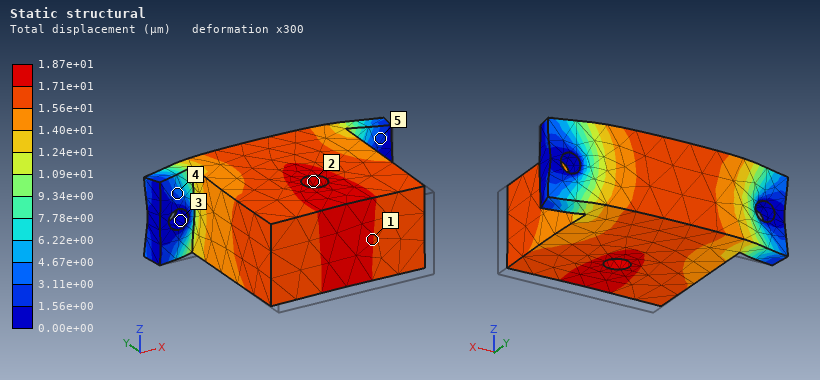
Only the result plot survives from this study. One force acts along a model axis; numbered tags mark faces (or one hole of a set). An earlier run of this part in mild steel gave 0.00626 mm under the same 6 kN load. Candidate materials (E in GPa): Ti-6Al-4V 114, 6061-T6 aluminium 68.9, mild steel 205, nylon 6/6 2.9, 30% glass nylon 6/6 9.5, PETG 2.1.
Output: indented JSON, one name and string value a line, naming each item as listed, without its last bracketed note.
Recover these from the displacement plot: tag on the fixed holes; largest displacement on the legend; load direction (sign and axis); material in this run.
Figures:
{
  "tag on the fixed holes": "3",
  "largest displacement on the legend": "1.87e+01 µm",
  "load direction": "+Y",
  "material in this run": "6061-T6 aluminium"
}
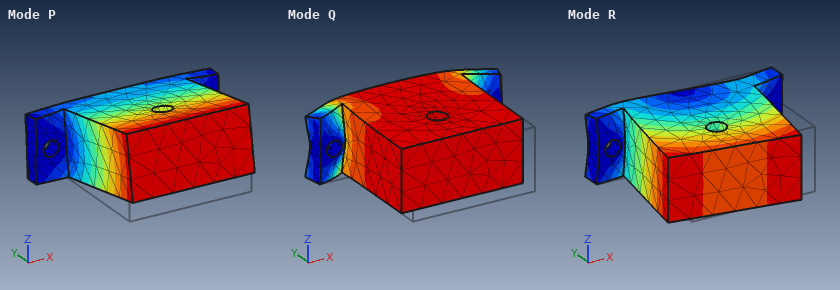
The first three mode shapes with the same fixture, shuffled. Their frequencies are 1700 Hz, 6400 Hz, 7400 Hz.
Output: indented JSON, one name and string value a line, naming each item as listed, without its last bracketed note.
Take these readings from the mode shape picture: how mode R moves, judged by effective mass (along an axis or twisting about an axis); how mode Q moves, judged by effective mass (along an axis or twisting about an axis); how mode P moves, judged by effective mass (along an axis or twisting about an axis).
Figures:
{
  "how mode R moves, judged by effective mass": "along X",
  "how mode Q moves, judged by effective mass": "along Y",
  "how mode P moves, judged by effective mass": "along Z"
}
